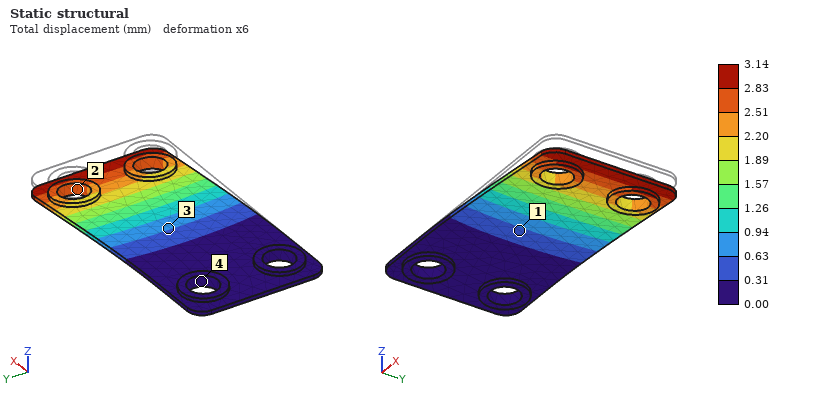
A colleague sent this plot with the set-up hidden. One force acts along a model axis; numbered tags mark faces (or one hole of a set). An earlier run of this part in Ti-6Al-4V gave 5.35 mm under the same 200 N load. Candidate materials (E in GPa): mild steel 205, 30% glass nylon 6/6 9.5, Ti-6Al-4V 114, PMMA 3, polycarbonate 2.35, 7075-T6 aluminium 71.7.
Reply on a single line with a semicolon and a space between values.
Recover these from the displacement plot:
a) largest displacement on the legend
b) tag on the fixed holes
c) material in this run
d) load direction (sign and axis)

3.14 mm; 4; mild steel; -Z
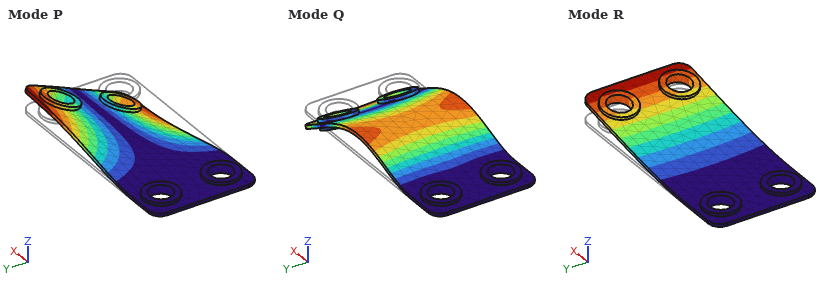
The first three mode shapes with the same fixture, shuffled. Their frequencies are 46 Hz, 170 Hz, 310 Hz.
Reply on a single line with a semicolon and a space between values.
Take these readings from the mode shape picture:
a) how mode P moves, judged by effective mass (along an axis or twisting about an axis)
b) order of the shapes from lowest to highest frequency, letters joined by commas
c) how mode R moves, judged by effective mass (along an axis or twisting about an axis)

twisting about X; R, P, Q; along Z
